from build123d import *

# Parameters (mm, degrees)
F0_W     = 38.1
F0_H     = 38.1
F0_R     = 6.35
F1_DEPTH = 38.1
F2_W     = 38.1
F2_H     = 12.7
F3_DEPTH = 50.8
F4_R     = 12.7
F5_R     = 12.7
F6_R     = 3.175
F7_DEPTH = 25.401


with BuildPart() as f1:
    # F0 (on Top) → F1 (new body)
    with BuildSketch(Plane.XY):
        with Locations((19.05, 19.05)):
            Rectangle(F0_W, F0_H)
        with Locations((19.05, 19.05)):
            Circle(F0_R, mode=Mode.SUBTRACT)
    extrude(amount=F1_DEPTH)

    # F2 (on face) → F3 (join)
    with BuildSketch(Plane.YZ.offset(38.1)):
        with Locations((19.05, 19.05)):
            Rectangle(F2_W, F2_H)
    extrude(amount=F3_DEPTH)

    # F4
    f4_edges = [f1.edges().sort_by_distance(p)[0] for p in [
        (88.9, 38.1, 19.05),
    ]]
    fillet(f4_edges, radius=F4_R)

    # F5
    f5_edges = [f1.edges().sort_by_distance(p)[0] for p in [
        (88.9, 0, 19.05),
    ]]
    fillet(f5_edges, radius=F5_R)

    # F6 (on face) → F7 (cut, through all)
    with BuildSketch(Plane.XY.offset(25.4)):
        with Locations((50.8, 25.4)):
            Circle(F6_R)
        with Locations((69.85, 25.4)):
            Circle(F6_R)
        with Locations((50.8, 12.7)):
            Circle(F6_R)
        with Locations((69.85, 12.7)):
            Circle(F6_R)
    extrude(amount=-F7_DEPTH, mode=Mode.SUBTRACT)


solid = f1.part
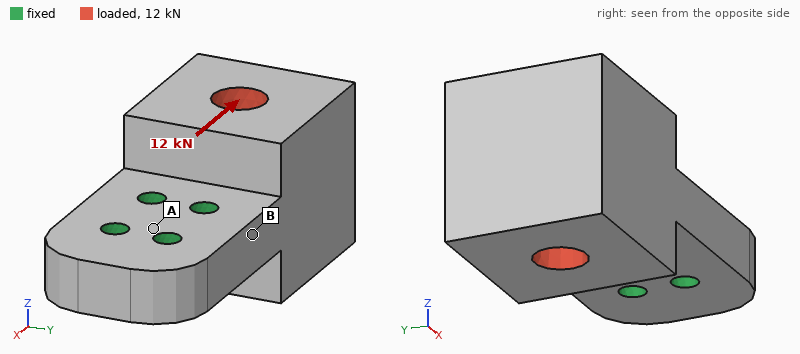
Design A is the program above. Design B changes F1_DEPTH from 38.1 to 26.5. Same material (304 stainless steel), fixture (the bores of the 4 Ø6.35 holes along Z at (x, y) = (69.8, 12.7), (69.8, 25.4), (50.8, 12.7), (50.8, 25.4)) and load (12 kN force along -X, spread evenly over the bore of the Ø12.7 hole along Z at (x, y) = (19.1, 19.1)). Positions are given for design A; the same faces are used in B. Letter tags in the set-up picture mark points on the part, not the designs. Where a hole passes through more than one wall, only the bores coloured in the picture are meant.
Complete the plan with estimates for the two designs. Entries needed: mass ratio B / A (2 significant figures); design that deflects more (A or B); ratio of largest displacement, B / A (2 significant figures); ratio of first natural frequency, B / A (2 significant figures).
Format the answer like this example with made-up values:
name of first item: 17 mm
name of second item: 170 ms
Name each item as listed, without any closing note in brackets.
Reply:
mass ratio B / A: 0.79
design that deflects more: B
ratio of largest displacement, B / A: 10
ratio of first natural frequency, B / A: 1.2
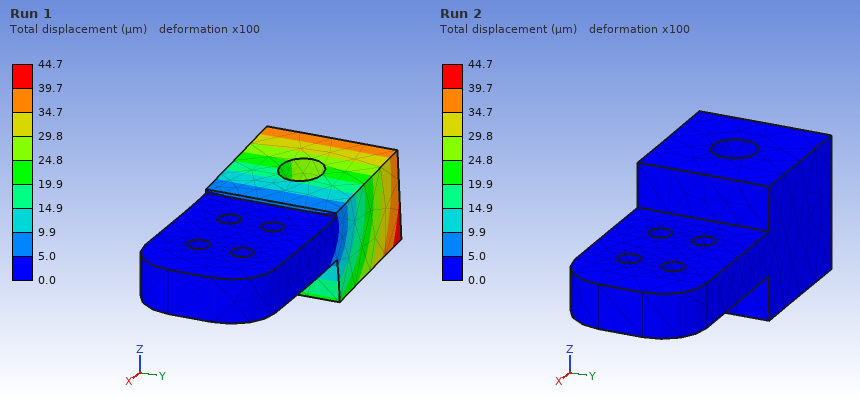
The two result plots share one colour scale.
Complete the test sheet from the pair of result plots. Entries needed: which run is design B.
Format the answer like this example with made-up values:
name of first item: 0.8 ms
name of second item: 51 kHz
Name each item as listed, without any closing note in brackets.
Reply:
which run is design B: Run 1
